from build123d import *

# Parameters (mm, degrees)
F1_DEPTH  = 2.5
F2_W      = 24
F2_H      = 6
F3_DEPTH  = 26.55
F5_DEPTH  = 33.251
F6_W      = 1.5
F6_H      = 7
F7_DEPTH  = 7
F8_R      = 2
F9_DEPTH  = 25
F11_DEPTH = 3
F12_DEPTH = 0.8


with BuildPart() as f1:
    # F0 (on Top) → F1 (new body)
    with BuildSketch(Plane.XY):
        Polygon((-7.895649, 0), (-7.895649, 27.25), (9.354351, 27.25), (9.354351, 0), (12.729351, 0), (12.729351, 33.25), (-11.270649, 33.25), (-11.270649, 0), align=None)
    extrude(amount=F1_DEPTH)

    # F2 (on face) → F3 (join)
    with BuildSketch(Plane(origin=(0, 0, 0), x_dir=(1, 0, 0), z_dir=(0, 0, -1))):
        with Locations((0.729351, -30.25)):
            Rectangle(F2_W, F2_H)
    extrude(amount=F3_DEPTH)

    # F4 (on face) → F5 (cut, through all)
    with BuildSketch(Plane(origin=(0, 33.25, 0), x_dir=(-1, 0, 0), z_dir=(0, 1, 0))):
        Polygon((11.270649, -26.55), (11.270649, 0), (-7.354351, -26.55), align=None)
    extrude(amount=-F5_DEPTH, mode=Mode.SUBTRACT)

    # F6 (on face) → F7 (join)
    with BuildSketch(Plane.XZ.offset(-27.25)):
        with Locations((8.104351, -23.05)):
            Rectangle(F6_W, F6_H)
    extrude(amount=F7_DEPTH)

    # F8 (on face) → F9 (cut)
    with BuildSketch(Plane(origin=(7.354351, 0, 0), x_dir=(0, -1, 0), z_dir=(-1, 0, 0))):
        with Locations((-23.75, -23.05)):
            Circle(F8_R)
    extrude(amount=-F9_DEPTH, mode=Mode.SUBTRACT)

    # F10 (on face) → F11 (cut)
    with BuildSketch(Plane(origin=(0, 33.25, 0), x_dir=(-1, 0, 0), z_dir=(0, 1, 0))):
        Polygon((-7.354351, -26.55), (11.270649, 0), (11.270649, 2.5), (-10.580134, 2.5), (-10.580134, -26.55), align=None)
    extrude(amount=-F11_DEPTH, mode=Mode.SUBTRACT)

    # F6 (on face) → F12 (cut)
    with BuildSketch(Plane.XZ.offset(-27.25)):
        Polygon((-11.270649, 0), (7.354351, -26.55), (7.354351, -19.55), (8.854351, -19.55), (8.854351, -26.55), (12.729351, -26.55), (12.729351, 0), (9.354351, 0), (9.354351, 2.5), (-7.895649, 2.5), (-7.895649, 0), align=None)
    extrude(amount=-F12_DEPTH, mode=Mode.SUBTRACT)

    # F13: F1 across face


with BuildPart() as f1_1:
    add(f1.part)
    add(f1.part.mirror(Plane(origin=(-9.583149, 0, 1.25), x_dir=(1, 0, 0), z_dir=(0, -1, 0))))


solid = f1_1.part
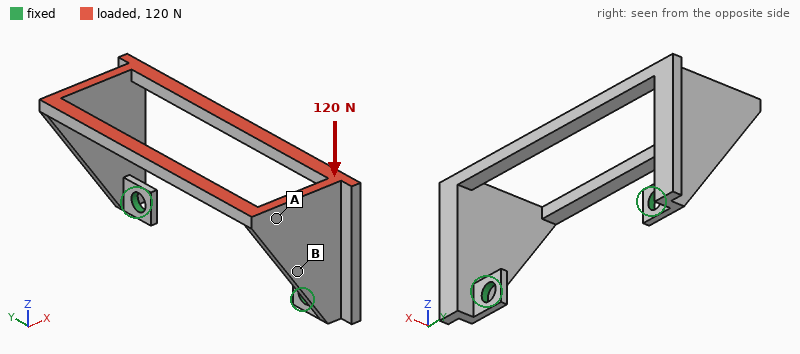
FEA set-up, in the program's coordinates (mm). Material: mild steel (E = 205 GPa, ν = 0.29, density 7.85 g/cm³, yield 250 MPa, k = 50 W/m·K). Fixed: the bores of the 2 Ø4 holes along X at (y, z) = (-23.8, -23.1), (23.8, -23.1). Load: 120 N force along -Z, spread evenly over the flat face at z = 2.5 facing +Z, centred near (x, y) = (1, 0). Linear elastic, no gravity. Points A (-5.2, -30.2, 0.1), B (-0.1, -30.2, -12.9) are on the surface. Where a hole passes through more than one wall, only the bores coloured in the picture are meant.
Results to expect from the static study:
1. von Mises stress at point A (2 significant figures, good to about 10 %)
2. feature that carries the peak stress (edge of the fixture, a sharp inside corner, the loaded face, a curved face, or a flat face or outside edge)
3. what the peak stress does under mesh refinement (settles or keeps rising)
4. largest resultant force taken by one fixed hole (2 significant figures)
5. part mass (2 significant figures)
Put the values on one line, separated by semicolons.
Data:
27 MPa; edge of the fixture; keeps rising; 62 N; 27 g
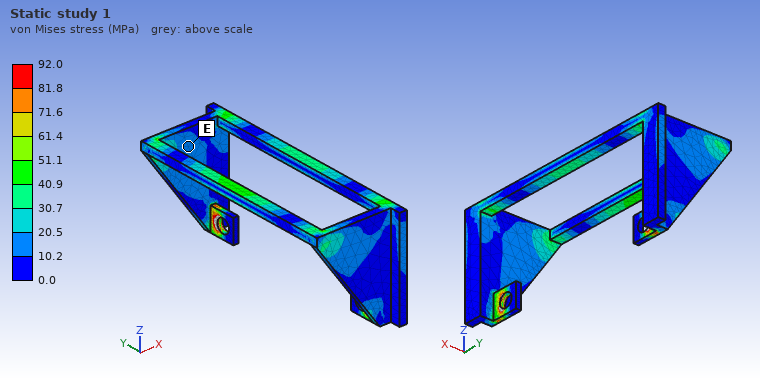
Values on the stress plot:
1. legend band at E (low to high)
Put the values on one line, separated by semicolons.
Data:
10.2 to 20.5 MPa
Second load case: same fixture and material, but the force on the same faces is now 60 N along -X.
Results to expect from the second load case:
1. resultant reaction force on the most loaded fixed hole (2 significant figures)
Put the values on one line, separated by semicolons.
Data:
30 N
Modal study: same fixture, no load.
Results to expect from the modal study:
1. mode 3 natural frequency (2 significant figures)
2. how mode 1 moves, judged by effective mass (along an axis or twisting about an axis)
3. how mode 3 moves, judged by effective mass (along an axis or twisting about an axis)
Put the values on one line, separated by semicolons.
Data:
2000 Hz; along X; along Y
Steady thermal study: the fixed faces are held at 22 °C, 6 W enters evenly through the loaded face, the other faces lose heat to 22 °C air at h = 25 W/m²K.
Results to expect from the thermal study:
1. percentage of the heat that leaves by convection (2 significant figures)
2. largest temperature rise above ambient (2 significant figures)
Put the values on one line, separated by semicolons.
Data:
47 %; 68 K
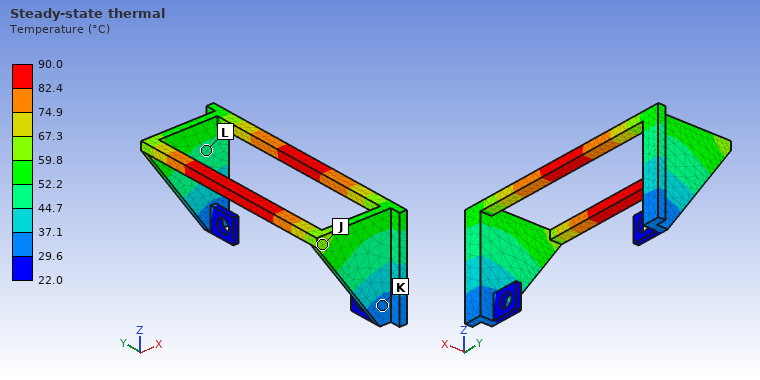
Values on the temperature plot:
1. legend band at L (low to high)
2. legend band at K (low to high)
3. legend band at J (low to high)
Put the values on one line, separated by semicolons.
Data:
44.7 to 52.2 °C; 29.6 to 37.1 °C; 59.8 to 67.3 °C
